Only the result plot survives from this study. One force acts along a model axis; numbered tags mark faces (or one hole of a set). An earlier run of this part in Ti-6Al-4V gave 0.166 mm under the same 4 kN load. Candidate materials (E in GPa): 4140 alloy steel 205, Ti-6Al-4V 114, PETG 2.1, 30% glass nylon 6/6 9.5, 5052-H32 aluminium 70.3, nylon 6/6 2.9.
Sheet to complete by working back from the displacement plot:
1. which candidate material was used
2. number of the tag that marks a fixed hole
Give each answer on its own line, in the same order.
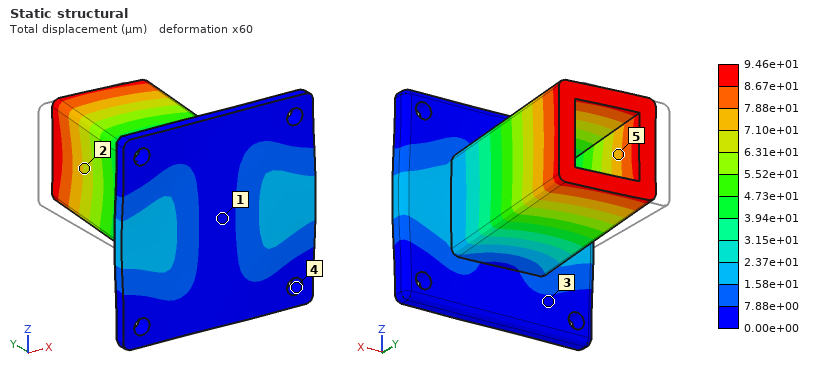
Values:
4140 alloy steel
4
